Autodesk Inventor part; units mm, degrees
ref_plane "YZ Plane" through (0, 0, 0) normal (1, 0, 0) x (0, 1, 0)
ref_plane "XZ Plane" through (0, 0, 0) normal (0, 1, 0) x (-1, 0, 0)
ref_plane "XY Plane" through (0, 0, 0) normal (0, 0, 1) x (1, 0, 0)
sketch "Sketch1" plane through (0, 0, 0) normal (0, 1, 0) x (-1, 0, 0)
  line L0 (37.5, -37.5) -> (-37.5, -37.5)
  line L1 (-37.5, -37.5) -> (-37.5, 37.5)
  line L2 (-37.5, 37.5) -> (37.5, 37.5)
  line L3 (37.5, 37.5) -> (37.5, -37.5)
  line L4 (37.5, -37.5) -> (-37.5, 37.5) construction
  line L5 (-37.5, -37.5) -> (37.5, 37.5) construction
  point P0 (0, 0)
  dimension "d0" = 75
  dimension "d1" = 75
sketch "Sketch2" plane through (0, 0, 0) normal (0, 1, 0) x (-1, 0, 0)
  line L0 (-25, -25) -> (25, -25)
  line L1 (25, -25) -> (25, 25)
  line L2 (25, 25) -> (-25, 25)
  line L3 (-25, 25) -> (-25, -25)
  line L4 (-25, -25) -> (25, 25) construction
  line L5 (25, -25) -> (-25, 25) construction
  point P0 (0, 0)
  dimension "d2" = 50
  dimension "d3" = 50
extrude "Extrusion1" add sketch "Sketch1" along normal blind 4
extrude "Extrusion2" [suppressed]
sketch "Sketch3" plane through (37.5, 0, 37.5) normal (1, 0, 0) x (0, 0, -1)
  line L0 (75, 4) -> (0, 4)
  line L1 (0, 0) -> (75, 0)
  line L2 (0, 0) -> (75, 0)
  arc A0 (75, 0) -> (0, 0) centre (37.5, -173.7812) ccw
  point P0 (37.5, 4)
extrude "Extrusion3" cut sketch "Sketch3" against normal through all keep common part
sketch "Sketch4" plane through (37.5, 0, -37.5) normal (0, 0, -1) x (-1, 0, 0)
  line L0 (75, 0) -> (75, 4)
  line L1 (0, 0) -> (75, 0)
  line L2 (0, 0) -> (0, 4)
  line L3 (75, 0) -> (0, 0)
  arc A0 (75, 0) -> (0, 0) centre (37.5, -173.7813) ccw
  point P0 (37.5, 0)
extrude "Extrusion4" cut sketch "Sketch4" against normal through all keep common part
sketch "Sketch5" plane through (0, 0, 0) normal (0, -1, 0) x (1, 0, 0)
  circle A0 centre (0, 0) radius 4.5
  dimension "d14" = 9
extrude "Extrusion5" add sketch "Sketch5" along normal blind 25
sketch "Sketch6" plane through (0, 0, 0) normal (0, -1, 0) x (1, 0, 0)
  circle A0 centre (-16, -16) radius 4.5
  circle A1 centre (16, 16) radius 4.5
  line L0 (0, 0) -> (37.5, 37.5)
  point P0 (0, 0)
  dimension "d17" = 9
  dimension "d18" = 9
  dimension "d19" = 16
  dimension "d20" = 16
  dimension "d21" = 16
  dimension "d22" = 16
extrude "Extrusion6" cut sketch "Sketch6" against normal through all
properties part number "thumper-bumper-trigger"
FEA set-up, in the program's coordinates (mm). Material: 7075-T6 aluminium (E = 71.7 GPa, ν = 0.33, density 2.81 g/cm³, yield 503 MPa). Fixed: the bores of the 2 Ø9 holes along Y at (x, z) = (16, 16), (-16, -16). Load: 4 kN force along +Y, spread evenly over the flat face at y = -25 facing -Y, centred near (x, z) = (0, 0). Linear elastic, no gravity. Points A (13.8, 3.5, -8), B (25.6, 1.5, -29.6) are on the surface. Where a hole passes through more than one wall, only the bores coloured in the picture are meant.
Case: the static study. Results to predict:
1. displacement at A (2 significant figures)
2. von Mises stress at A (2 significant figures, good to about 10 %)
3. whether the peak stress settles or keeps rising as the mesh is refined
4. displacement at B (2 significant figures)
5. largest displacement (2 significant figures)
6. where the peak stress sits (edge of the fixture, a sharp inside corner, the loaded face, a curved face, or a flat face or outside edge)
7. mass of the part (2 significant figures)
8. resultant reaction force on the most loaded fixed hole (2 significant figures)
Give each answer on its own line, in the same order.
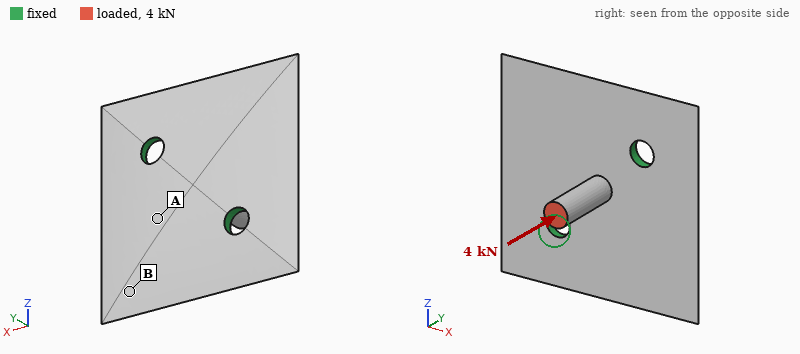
0.12 mm
87 MPa
keeps rising
0.16 mm
0.20 mm
edge of the fixture
35 g
2.1 kN
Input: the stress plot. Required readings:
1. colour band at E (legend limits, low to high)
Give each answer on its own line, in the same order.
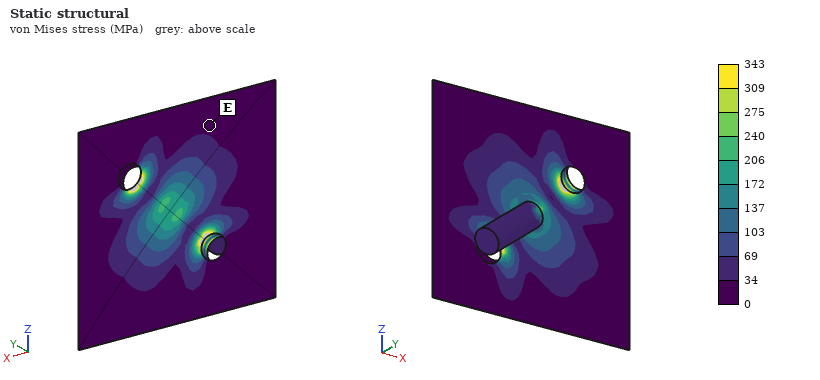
0 to 34 MPa
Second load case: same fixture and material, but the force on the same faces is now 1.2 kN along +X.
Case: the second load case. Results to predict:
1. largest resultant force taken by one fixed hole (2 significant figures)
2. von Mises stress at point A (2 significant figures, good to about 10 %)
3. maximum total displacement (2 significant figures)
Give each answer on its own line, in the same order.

980 N
82 MPa
0.72 mm
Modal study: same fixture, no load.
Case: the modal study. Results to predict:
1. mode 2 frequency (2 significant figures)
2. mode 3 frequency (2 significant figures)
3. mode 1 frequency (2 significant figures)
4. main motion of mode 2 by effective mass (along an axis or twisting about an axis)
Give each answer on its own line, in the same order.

2600 Hz
5300 Hz
2100 Hz
along Y
